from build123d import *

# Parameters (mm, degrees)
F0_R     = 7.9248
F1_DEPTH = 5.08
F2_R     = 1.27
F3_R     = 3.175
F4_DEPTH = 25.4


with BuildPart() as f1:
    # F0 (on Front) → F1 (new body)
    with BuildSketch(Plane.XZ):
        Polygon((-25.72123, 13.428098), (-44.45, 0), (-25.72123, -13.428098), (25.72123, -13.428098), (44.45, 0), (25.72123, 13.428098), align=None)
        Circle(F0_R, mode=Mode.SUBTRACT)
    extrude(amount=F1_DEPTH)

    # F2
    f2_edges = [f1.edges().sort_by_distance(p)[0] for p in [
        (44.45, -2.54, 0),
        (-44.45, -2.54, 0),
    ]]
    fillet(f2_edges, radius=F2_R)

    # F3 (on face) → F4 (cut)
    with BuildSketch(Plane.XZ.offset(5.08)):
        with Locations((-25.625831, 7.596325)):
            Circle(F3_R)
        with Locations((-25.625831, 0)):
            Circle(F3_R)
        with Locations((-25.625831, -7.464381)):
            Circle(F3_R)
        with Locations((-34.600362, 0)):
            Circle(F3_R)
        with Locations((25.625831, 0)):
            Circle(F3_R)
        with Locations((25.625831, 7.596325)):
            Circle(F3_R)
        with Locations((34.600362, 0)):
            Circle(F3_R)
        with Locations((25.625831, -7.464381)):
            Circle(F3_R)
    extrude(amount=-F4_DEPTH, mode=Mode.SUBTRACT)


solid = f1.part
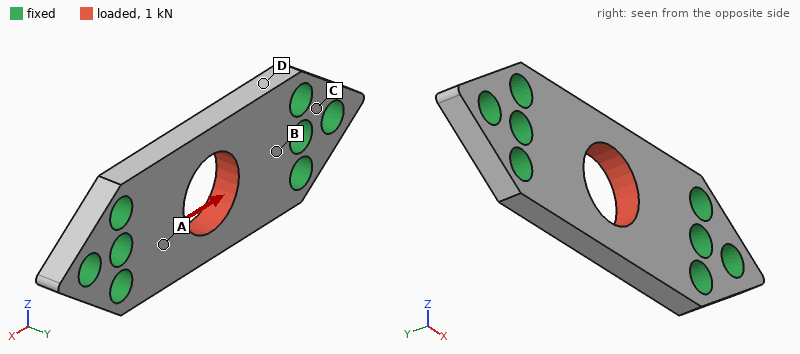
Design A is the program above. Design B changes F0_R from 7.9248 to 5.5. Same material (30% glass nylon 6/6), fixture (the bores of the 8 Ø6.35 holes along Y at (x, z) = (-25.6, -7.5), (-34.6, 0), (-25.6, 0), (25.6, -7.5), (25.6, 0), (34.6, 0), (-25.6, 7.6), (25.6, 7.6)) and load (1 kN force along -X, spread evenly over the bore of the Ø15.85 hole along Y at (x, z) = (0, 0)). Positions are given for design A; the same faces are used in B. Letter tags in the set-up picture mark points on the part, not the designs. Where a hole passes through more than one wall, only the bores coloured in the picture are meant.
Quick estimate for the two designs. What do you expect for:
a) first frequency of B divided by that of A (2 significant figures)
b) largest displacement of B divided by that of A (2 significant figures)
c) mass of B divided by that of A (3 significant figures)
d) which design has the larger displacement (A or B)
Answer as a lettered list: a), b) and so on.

a) 0.94
b) 1.1
c) 1.07
d) B
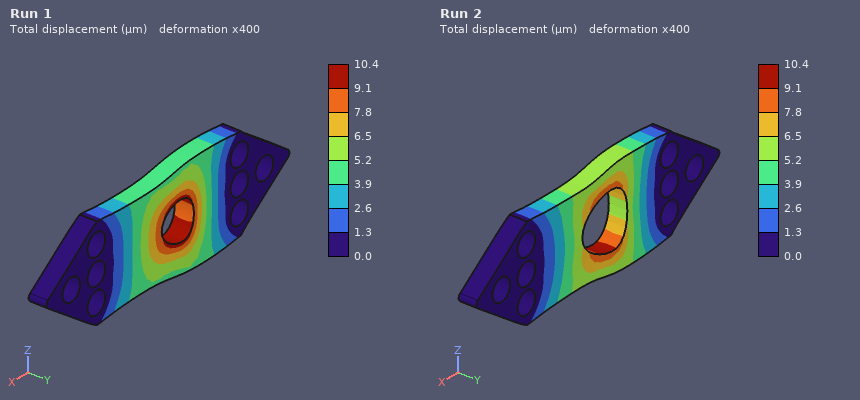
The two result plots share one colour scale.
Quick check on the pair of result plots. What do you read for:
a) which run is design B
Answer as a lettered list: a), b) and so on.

a) Run 1
